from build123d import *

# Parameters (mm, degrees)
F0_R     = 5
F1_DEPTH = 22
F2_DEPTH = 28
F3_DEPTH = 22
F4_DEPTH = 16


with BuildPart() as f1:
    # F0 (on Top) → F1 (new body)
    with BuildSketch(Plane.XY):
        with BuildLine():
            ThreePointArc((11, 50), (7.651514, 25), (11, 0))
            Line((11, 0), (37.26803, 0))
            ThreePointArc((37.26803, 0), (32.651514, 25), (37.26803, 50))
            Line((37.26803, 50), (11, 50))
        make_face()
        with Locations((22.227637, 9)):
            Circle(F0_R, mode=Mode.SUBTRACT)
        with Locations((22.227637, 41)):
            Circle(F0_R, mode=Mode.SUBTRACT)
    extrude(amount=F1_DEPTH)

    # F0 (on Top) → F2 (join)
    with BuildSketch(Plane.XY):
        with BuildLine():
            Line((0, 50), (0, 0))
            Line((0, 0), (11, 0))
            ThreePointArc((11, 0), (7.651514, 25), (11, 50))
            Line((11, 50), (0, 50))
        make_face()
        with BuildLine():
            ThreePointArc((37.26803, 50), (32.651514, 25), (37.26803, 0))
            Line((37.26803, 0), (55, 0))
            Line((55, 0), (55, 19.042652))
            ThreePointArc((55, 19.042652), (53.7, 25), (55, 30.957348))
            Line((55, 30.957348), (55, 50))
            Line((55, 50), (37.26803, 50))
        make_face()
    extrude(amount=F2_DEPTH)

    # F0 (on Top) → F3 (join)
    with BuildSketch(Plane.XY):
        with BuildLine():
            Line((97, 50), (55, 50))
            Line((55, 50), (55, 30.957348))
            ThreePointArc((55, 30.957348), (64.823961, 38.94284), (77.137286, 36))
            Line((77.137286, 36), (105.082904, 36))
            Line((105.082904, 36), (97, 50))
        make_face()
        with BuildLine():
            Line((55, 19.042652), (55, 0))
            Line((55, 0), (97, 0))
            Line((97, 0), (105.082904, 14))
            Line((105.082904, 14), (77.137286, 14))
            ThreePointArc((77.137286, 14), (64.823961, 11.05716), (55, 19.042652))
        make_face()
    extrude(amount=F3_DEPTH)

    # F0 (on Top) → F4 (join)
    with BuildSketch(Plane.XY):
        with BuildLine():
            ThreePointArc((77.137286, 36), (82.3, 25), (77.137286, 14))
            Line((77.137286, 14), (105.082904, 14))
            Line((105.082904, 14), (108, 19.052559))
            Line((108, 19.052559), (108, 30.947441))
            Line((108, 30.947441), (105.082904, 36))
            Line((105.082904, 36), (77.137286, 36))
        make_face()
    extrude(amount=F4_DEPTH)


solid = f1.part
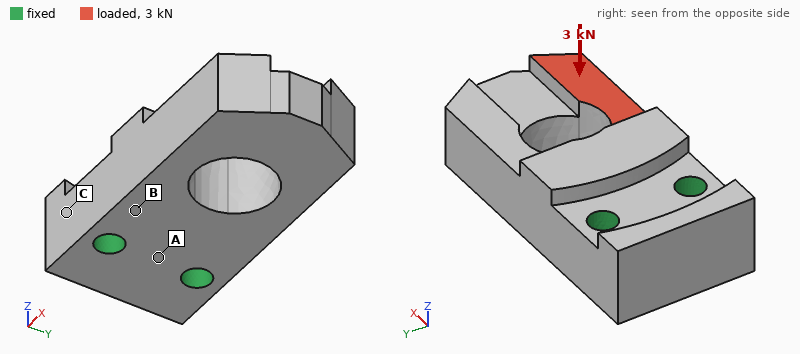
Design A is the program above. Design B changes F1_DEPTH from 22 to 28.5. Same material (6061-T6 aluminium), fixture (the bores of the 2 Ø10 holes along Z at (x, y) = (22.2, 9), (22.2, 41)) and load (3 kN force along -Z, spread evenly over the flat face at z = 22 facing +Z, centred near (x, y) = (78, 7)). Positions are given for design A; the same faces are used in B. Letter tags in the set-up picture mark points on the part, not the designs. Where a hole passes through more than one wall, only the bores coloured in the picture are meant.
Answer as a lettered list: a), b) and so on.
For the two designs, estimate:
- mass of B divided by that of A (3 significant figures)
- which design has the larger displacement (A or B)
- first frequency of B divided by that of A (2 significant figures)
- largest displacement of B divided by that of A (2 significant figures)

a) 1.07
b) A
c) 1.2
d) 0.76
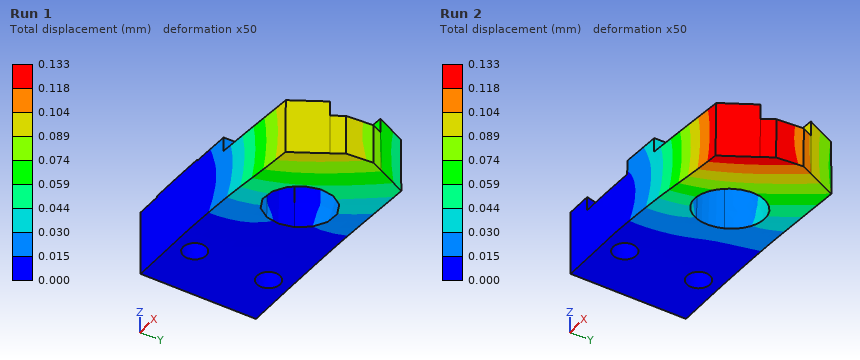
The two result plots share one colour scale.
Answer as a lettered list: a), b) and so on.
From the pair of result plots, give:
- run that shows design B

a) Run 1
